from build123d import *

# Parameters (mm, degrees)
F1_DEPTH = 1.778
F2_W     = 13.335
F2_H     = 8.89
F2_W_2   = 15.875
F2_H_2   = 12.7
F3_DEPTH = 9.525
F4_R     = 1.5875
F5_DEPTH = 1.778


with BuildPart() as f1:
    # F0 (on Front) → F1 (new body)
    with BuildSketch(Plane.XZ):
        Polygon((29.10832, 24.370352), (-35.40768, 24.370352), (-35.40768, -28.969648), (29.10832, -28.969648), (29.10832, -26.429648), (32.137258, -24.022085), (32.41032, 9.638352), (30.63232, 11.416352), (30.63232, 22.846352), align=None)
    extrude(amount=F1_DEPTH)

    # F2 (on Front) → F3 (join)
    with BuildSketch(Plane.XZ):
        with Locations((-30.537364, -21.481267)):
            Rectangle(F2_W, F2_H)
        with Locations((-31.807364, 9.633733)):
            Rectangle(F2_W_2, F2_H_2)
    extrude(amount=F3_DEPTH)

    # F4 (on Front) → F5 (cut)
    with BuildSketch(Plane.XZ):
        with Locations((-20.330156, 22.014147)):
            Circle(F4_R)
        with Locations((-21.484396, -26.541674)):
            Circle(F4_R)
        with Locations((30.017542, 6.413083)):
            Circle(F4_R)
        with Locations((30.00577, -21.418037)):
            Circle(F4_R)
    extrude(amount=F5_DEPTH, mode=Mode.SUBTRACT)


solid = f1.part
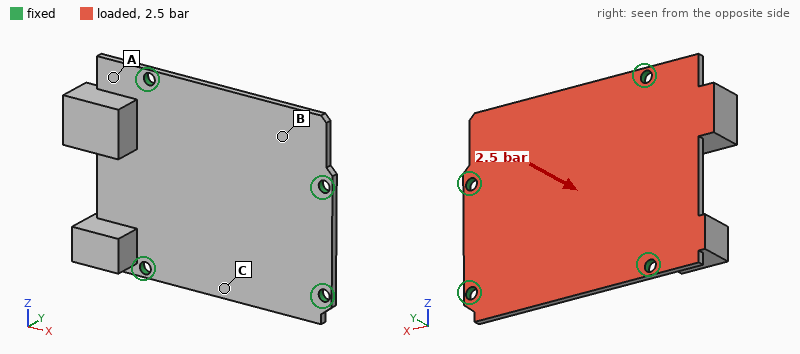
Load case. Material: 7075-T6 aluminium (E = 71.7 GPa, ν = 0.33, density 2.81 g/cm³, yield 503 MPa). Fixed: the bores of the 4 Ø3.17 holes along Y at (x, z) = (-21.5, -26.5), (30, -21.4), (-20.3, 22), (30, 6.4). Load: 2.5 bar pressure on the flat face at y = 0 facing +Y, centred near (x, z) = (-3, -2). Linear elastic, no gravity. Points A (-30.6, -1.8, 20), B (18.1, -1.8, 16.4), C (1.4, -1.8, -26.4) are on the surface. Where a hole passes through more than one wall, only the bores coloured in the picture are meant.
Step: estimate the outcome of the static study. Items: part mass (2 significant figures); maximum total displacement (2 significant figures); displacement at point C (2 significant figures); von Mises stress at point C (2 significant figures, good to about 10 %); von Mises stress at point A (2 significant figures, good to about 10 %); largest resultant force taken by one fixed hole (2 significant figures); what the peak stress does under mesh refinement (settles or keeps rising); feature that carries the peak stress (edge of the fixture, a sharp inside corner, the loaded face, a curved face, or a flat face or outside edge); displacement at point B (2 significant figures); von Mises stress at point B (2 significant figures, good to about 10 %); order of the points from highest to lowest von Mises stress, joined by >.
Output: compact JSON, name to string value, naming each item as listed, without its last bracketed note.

{"part mass": "25 g", "maximum total displacement": "0.21 mm", "displacement at point C": "0.15 mm", "von Mises stress at point C": "59 MPa", "von Mises stress at point A": "17 MPa", "largest resultant force taken by one fixed hole": "270 N", "what the peak stress does under mesh refinement": "keeps rising", "feature that carries the peak stress": "edge of the fixture", "displacement at point B": "0.13 mm", "von Mises stress at point B": "34 MPa", "order of the points from highest to lowest von Mises stress, joined by >": "C > B > A"}
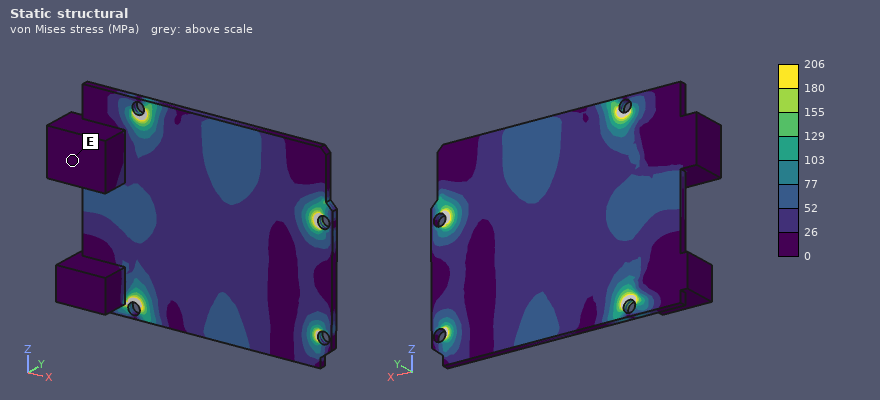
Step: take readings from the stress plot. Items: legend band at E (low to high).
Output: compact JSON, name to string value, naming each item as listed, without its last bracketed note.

{"legend band at E": "0 to 26 MPa"}
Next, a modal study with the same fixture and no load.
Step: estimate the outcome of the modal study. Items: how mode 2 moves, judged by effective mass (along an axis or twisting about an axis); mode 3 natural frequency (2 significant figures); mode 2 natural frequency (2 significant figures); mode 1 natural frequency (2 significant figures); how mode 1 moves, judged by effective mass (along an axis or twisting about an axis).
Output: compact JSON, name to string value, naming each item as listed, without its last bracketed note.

{"how mode 2 moves, judged by effective mass": "along Y", "mode 3 natural frequency": "3500 Hz", "mode 2 natural frequency": "2800 Hz", "mode 1 natural frequency": "1900 Hz", "how mode 1 moves, judged by effective mass": "along Y"}
